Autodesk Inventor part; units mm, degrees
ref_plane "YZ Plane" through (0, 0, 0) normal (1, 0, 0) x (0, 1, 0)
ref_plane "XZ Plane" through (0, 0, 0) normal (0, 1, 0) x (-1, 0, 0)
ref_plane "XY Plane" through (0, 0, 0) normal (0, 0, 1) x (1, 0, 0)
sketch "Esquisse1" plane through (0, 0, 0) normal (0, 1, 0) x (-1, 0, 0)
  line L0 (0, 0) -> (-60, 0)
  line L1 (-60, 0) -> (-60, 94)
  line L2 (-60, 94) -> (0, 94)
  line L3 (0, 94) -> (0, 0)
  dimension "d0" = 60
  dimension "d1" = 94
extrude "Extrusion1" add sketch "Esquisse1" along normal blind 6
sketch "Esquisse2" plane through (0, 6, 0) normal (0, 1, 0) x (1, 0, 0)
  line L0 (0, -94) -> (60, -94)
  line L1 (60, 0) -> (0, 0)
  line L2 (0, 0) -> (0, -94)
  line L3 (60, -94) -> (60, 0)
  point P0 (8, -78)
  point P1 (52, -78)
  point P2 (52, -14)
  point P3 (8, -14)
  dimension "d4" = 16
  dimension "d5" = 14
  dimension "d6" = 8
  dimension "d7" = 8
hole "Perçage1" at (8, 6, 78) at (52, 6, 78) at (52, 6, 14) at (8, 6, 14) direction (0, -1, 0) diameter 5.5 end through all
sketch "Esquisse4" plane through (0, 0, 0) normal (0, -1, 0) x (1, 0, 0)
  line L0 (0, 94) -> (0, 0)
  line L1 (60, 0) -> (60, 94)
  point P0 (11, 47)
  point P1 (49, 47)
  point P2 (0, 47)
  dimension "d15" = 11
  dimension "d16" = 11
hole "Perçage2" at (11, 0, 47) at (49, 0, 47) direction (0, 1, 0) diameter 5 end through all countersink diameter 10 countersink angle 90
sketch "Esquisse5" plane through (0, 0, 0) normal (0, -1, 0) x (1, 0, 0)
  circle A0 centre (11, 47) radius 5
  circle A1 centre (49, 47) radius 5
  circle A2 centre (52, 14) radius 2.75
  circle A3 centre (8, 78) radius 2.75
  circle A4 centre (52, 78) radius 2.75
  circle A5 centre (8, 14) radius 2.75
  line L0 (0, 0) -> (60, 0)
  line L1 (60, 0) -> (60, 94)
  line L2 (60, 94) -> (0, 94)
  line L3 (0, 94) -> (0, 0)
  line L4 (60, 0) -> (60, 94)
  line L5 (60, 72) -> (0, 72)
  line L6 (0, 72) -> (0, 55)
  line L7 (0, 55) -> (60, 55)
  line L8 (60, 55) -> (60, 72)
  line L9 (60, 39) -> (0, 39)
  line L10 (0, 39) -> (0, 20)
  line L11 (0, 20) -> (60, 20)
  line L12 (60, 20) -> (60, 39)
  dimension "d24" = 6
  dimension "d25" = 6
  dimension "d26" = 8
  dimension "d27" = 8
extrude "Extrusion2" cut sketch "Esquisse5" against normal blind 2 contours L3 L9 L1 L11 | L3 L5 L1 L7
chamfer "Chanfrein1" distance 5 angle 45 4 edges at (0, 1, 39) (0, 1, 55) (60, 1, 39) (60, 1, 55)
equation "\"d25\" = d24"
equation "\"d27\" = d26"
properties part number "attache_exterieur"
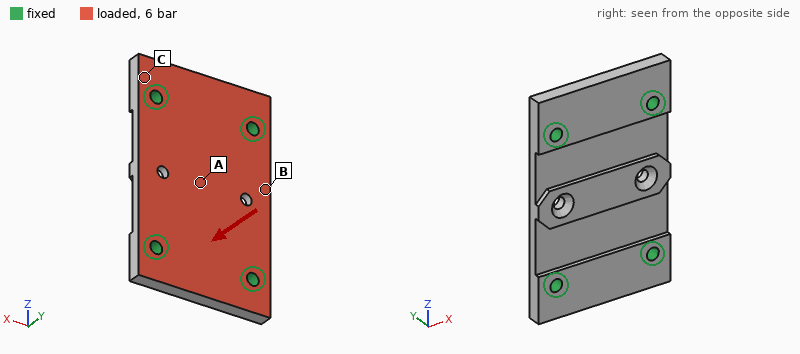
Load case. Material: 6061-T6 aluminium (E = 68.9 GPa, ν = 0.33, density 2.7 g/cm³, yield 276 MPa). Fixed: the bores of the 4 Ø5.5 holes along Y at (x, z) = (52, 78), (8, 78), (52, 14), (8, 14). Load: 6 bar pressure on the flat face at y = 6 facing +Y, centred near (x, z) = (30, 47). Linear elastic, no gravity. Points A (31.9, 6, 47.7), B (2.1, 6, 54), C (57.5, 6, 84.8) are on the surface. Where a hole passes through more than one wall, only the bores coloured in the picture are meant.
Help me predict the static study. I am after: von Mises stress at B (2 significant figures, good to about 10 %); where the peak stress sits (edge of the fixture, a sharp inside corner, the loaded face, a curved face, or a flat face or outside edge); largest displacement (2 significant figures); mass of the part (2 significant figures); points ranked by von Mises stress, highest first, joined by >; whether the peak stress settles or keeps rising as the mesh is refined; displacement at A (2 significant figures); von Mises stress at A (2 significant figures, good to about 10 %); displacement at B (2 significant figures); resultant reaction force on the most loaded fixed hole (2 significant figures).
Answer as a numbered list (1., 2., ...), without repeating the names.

1. 25 MPa
2. edge of the fixture
3. 44 µm
4. 77 g
5. B > A > C
6. keeps rising
7. 44 µm
8. 15 MPa
9. 37 µm
10. 850 N
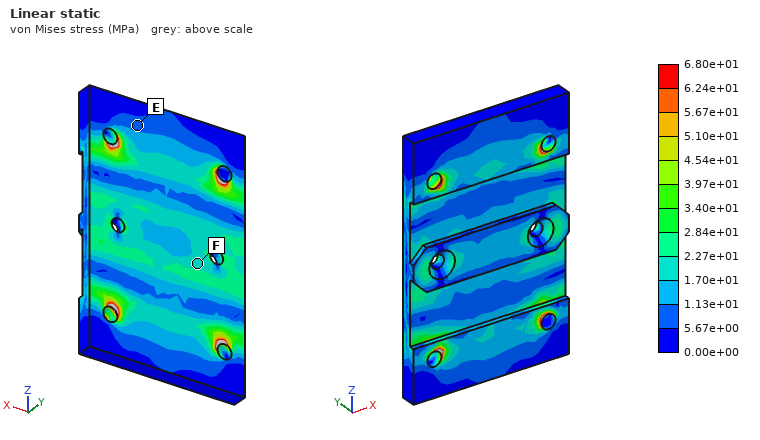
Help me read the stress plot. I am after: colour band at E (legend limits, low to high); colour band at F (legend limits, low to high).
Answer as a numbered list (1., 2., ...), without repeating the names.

1. 5.67e+00 to 1.13e+01 MPa
2. 1.70e+01 to 2.27e+01 MPa
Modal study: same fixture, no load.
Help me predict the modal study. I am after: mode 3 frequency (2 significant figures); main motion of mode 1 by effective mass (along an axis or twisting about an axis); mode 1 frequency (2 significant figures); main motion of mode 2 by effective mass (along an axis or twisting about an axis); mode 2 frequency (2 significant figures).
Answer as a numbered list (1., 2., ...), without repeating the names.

1. 11 kHz
2. along Y
3. 5700 Hz
4. twisting about Z
5. 7200 Hz
